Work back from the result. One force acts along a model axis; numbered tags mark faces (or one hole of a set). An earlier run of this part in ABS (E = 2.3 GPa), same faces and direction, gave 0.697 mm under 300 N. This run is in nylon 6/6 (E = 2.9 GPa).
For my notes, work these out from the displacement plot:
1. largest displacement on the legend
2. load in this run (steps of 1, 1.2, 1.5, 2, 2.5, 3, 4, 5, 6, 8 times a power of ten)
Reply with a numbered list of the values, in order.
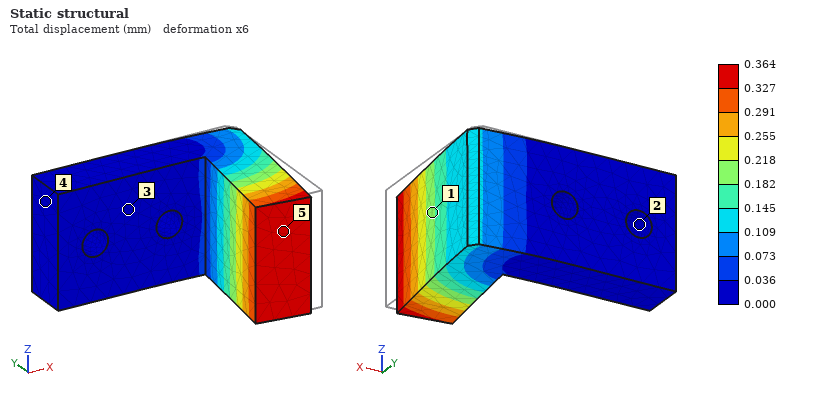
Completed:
1. 0.364 mm
2. 200 N
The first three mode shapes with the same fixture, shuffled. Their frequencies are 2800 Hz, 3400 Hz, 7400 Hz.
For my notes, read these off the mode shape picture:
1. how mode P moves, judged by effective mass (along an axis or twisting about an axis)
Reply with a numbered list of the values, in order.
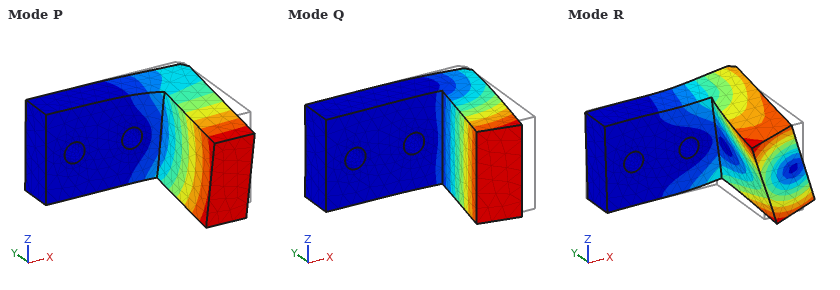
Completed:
1. along Z
